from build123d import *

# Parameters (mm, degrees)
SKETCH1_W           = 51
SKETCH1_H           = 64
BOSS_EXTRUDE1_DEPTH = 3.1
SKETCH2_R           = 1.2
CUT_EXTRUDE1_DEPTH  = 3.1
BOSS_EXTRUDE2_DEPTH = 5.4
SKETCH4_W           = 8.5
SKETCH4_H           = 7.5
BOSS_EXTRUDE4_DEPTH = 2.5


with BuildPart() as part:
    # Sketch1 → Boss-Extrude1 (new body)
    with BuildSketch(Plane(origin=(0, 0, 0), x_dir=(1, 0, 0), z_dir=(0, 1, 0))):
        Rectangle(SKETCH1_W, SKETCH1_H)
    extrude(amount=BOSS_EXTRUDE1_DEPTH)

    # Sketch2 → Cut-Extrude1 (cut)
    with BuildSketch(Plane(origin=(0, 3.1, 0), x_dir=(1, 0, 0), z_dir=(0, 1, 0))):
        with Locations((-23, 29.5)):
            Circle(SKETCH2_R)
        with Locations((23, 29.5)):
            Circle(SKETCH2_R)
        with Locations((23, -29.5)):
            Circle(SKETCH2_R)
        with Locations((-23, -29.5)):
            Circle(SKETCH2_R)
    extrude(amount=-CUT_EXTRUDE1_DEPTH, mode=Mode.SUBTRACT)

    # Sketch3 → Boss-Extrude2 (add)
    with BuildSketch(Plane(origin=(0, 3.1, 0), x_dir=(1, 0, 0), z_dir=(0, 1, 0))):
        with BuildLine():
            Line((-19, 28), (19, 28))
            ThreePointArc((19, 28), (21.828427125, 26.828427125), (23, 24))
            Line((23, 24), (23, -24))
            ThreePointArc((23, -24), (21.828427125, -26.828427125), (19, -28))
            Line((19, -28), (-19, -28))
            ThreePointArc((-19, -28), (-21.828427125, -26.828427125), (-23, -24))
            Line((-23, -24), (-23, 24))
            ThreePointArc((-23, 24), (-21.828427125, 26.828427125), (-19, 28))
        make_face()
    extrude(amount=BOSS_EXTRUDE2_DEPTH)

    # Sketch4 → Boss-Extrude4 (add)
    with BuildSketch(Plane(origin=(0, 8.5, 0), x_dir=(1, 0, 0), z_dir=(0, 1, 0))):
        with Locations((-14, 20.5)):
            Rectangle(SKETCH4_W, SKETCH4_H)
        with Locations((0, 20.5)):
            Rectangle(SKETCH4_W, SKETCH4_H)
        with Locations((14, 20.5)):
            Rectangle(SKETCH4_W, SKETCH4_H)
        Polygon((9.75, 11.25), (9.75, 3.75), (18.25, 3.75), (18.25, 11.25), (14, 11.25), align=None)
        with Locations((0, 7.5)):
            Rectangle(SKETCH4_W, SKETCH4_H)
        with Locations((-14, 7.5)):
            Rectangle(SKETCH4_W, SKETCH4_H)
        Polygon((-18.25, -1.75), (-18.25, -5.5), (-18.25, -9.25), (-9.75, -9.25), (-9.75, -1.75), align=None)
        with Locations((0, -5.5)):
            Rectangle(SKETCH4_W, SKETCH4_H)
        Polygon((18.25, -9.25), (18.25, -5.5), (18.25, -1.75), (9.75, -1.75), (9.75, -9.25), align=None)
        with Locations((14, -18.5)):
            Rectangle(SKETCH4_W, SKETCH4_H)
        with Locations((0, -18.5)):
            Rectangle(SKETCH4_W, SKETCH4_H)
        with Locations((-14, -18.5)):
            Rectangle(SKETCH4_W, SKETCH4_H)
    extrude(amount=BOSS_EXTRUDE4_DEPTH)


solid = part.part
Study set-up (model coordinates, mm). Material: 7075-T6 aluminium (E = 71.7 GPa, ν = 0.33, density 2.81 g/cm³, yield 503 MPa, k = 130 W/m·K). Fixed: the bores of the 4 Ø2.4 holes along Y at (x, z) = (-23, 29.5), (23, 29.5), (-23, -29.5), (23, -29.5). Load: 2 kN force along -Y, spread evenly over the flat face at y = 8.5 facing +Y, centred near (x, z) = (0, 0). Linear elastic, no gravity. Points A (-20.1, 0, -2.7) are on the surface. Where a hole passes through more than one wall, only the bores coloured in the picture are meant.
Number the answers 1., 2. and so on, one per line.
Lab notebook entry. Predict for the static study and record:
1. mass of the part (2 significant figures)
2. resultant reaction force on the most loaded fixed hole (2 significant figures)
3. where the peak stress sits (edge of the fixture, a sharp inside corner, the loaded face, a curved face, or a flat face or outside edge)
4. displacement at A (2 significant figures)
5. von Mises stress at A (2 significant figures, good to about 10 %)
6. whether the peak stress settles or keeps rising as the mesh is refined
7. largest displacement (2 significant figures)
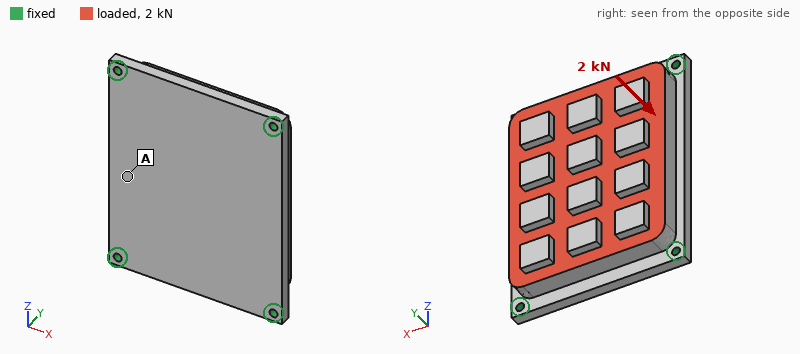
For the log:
1. 73 g
2. 750 N
3. edge of the fixture
4. 25 µm
5. 15 MPa
6. keeps rising
7. 26 µm
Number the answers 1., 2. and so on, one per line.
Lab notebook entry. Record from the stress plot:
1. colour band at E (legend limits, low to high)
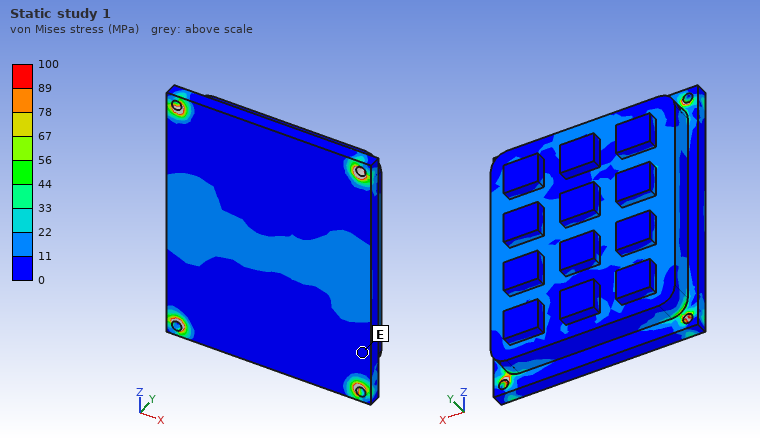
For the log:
1. 0 to 11 MPa
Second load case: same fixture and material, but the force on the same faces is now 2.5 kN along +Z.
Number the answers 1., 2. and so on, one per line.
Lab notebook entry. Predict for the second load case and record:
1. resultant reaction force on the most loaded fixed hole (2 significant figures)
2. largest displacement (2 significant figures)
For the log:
1. 690 N
2. 5.9 µm
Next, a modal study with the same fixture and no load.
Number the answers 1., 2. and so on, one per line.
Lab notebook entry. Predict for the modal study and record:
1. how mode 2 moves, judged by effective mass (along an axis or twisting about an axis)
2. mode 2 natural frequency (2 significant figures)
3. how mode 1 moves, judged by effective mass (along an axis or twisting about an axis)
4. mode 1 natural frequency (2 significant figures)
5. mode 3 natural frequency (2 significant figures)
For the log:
1. twisting about Z
2. 9800 Hz
3. along Y
4. 5800 Hz
5. 11 kHz
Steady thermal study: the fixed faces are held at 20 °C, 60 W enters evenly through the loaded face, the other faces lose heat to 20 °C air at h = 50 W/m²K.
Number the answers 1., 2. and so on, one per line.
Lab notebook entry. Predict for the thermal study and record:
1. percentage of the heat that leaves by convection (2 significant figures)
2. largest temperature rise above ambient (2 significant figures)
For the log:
1. 14 %
2. 27 K
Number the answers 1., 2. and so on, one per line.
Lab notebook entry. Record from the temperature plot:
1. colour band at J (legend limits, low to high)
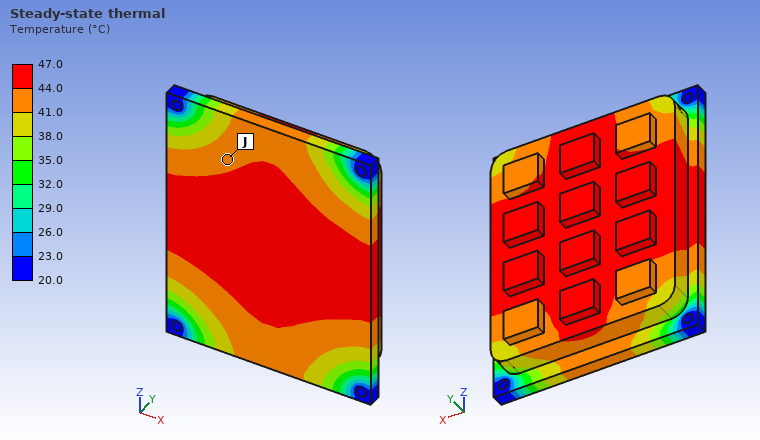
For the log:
1. 41.0 to 44.0 °C
